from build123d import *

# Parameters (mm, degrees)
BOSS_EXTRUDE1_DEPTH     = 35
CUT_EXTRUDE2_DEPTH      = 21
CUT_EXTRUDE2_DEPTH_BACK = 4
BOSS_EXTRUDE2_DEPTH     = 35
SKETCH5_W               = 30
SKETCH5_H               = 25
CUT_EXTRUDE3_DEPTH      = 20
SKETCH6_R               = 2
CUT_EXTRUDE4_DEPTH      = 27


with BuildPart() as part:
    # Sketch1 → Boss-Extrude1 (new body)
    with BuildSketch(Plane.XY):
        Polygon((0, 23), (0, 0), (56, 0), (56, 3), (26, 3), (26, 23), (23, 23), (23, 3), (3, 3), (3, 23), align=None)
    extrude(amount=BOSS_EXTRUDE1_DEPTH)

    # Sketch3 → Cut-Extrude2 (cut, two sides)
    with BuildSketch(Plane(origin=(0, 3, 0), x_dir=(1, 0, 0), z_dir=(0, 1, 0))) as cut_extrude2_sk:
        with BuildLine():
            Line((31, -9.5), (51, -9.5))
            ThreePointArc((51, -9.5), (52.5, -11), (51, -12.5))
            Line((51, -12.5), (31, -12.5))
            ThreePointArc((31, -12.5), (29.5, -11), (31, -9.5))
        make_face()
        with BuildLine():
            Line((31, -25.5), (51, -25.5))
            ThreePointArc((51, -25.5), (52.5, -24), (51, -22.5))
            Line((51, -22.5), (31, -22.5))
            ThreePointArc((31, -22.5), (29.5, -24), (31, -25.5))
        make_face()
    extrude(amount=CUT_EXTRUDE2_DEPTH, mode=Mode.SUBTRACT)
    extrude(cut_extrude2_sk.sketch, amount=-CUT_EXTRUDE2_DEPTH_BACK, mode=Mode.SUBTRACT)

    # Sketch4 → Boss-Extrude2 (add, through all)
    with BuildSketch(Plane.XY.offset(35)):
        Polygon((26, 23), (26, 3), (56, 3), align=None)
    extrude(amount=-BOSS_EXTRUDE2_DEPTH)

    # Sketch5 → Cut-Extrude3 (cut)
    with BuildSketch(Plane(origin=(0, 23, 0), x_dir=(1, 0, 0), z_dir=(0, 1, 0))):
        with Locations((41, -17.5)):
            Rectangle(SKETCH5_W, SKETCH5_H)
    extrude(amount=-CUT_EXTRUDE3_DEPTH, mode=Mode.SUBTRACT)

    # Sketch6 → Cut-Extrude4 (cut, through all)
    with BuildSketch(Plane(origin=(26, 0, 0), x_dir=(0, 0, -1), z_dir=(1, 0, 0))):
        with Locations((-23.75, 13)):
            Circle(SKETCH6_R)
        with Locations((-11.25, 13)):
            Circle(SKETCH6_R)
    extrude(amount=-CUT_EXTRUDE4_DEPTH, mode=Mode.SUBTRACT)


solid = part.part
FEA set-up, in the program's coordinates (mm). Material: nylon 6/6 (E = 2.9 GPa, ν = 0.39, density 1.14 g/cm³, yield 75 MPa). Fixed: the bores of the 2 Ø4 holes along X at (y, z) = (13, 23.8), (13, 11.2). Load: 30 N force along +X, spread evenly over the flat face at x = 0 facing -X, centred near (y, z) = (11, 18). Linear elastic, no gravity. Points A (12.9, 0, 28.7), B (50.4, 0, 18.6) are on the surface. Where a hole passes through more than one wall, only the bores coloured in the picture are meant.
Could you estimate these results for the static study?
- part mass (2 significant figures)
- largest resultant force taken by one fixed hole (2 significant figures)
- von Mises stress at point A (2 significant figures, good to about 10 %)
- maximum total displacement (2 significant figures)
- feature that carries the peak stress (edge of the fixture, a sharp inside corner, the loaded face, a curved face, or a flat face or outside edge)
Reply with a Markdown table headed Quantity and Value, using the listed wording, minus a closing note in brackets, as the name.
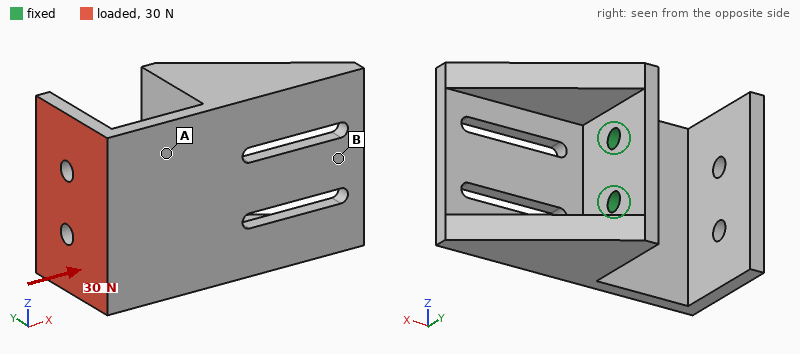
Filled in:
| Quantity | Value |
|---|---|
| part mass | 14 g |
| largest resultant force taken by one fixed hole | 15 N |
| von Mises stress at point A | 4.9 MPa |
| maximum total displacement | 0.82 mm |
| feature that carries the peak stress | a flat face or outside edge |
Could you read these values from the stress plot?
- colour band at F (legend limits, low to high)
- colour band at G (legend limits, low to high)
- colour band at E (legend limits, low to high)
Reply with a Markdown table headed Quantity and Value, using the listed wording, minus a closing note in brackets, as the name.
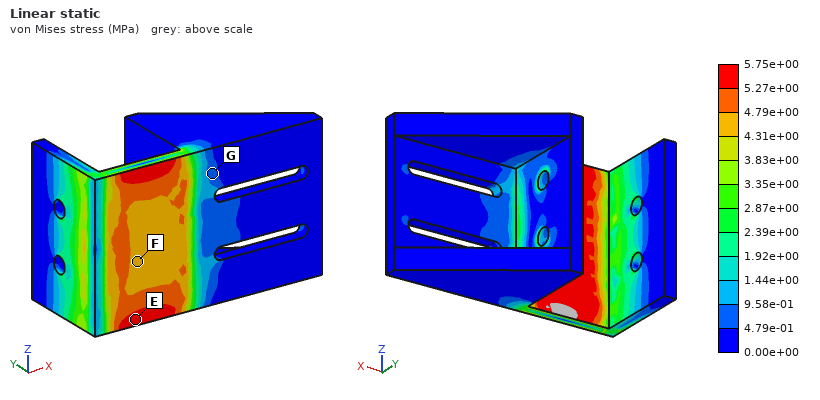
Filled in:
| Quantity | Value |
|---|---|
| colour band at F | 4.31e+00 to 4.79e+00 MPa |
| colour band at G | 4.79e-01 to 9.58e-01 MPa |
| colour band at E | 5.27e+00 to 5.75e+00 MPa |
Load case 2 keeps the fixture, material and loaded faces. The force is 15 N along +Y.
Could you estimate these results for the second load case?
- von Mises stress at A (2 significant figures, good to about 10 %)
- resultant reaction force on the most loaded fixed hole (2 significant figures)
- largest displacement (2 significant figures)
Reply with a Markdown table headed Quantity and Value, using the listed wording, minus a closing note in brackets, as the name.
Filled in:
| Quantity | Value |
|---|---|
| von Mises stress at A | 3.4 MPa |
| resultant reaction force on the most loaded fixed hole | 7.5 N |
| largest displacement | 0.65 mm |
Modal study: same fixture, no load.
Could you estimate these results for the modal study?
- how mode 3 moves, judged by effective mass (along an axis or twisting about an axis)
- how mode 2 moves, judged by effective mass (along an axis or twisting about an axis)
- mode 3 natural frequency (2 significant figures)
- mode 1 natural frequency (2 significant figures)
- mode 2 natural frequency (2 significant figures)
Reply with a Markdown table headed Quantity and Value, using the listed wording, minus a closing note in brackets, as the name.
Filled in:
| Quantity | Value |
|---|---|
| how mode 3 moves, judged by effective mass | along X |
| how mode 2 moves, judged by effective mass | twisting about Y |
| mode 3 natural frequency | 920 Hz |
| mode 1 natural frequency | 470 Hz |
| mode 2 natural frequency | 720 Hz |
